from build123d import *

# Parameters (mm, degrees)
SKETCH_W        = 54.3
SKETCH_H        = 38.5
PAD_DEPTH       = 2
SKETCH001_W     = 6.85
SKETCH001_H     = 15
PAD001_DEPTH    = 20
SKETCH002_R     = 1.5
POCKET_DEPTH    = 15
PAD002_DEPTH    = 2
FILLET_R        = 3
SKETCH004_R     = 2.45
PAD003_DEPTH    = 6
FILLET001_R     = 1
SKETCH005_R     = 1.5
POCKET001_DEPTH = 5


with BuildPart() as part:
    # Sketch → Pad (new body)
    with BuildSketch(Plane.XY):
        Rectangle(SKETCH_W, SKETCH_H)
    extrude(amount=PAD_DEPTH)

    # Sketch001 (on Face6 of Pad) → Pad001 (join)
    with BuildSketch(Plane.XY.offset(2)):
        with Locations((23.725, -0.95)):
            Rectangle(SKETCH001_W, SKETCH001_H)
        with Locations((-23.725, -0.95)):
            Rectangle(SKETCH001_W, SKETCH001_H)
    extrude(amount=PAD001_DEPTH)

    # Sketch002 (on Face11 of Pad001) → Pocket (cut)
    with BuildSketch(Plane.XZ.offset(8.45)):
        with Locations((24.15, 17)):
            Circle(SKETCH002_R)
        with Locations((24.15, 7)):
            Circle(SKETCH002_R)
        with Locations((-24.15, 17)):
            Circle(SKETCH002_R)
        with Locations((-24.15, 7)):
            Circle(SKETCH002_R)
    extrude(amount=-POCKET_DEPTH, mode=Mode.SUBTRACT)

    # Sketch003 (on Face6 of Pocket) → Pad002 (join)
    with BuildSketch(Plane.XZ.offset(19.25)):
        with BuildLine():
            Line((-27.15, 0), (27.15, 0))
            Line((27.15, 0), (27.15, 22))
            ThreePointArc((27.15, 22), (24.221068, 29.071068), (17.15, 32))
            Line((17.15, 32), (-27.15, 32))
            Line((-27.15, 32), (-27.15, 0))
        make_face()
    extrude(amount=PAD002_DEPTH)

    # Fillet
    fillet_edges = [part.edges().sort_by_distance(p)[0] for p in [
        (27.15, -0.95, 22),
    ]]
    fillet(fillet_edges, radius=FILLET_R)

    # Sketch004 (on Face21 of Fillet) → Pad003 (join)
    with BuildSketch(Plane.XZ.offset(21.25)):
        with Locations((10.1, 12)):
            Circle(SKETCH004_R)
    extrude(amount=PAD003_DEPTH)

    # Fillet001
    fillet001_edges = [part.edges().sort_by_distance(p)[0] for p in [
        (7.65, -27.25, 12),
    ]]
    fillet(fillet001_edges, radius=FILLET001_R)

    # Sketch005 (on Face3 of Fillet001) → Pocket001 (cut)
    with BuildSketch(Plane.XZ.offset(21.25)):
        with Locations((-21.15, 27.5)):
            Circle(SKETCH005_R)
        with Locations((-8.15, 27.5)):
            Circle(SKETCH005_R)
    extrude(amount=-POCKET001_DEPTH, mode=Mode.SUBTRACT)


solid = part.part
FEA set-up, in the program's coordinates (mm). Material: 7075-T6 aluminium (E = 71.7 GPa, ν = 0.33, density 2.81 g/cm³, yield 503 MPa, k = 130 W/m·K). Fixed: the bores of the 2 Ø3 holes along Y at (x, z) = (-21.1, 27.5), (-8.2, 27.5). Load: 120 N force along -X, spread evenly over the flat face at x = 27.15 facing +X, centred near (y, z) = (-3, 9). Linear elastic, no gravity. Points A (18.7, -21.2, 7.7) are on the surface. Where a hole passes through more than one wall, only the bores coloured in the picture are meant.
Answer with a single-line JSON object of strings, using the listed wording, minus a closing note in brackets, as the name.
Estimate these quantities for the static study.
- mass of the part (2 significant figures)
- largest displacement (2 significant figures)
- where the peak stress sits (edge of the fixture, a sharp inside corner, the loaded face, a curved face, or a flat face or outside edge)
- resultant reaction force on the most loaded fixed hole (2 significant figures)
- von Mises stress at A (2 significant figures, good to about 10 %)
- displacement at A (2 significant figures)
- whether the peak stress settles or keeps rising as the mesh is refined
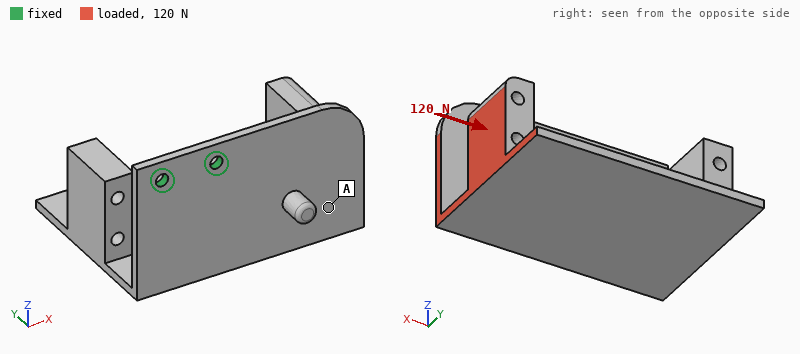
{"mass of the part": "32 g", "largest displacement": "0.80 mm", "where the peak stress sits": "edge of the fixture", "resultant reaction force on the most loaded fixed hole": "190 N", "von Mises stress at A": "9.1 MPa", "displacement at A": "0.36 mm", "whether the peak stress settles or keeps rising as the mesh is refined": "keeps rising"}
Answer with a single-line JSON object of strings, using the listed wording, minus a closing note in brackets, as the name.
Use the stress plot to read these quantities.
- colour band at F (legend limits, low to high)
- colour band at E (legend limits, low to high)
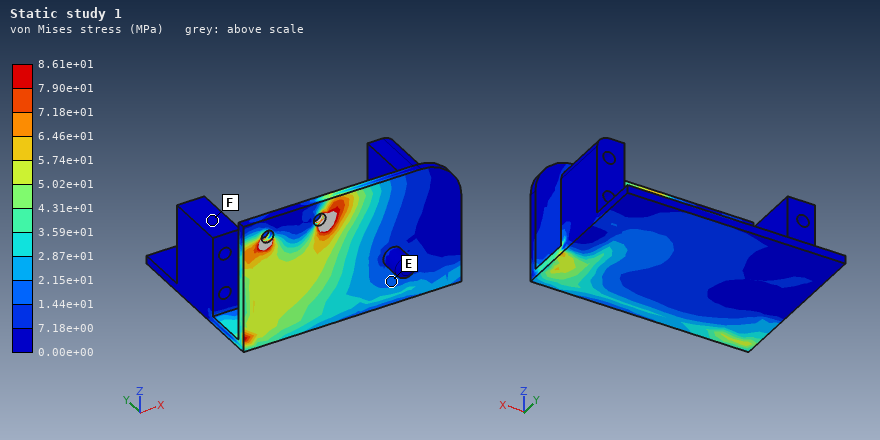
{"colour band at F": "0.00e+00 to 7.18e+00 MPa", "colour band at E": "1.44e+01 to 2.15e+01 MPa"}
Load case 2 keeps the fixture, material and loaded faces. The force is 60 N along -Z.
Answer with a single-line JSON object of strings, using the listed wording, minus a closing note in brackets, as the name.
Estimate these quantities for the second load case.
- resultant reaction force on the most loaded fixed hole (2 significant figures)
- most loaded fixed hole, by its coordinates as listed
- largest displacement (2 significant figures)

{"resultant reaction force on the most loaded fixed hole": "190 N", "most loaded fixed hole, by its coordinates as listed": "(-8.2, 27.5)", "largest displacement": "0.84 mm"}
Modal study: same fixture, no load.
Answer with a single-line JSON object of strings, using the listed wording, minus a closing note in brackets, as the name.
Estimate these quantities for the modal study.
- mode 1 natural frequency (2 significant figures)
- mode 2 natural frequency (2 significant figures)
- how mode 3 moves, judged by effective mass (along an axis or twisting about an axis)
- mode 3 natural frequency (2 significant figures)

{"mode 1 natural frequency": "340 Hz", "mode 2 natural frequency": "450 Hz", "how mode 3 moves, judged by effective mass": "along Y", "mode 3 natural frequency": "900 Hz"}
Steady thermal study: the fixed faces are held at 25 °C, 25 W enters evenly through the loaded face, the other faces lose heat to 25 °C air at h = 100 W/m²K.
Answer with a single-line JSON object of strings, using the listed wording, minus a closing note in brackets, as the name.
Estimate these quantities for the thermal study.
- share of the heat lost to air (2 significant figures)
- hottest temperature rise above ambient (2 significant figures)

{"share of the heat lost to air": "80 %", "hottest temperature rise above ambient": "57 K"}
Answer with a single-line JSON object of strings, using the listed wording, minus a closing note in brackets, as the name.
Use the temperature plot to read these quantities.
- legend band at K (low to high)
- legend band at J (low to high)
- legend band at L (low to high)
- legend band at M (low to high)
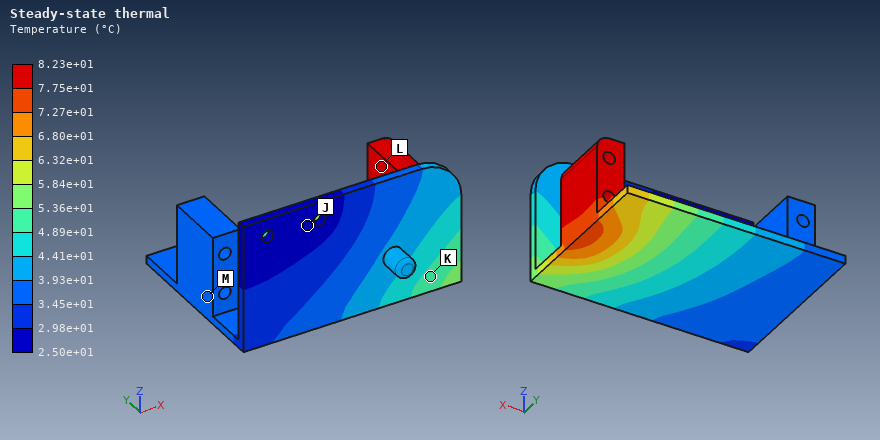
{"legend band at K": "4.89e+01 to 5.36e+01 °C", "legend band at J": "2.50e+01 to 2.98e+01 °C", "legend band at L": "7.75e+01 to 8.23e+01 °C", "legend band at M": "3.45e+01 to 3.93e+01 °C"}
